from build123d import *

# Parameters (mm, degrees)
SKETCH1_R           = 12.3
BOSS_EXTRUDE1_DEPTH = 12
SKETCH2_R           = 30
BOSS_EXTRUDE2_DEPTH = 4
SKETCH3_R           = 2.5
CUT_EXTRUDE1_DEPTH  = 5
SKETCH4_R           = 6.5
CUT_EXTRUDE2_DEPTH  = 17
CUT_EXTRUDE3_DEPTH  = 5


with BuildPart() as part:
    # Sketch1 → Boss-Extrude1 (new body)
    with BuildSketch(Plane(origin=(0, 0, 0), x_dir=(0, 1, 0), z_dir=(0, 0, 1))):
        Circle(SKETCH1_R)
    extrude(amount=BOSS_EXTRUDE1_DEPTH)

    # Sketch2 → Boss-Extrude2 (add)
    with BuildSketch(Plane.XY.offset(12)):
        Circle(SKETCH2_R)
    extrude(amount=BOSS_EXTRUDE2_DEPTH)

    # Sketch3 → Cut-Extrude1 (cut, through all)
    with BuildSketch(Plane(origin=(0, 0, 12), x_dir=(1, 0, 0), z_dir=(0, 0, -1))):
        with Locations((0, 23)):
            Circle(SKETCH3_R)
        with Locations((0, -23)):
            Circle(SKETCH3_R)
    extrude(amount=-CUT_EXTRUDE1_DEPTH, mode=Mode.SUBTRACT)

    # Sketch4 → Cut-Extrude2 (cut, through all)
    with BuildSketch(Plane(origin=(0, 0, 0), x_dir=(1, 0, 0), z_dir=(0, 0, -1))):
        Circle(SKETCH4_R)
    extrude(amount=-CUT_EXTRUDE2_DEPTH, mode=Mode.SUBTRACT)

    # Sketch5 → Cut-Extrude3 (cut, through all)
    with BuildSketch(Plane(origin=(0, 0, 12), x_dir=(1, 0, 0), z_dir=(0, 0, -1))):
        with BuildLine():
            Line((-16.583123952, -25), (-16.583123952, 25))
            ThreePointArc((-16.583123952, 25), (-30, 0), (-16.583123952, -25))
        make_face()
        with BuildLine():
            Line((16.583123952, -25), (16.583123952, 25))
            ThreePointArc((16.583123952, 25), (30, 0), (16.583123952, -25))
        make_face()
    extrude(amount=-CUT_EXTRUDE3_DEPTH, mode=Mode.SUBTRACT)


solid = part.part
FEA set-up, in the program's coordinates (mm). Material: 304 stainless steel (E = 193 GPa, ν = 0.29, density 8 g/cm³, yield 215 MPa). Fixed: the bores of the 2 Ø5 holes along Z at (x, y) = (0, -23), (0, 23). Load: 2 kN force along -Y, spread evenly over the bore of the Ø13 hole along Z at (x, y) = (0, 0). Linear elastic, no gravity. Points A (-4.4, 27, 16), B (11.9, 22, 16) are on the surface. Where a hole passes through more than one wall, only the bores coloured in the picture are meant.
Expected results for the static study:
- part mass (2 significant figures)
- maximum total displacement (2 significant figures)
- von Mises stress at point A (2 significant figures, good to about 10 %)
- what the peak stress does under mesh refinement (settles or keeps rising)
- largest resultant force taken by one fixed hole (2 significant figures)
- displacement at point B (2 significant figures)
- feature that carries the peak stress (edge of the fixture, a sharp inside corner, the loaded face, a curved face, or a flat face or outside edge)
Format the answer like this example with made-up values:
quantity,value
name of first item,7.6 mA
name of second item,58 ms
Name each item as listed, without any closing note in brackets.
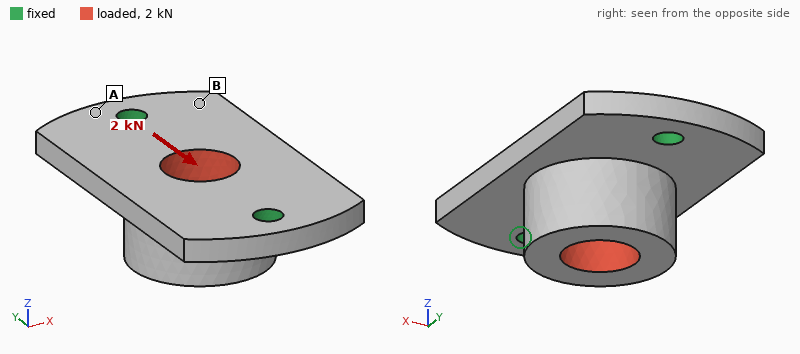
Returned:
quantity,value
part mass,88 g
maximum total displacement,5.2 µm
von Mises stress at point A,12 MPa
what the peak stress does under mesh refinement,keeps rising
largest resultant force taken by one fixed hole,1.1 kN
displacement at point B,1.3 µm
feature that carries the peak stress,edge of the fixture
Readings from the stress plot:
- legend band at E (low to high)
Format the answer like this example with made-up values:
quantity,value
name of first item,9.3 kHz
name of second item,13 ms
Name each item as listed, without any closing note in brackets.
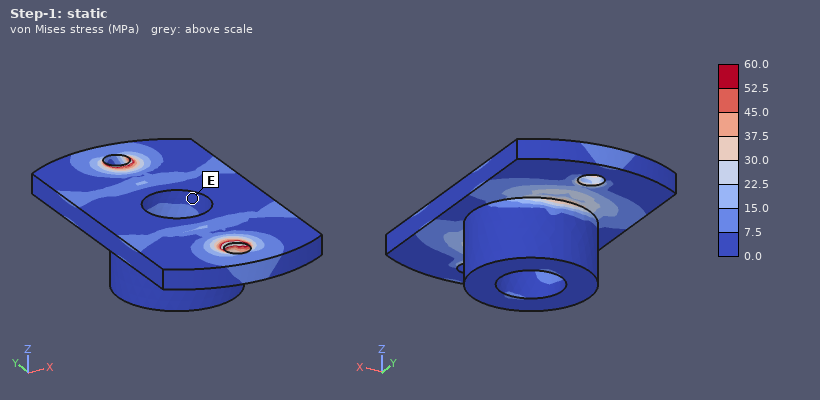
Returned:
quantity,value
legend band at E,0.0 to 7.5 MPa
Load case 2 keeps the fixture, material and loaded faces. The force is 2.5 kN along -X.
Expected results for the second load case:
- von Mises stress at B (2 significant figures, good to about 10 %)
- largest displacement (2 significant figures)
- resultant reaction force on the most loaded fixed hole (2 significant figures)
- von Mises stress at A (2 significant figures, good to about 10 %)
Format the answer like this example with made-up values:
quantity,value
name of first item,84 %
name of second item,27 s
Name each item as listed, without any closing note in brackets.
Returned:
quantity,value
von Mises stress at B,22 MPa
largest displacement,40 µm
resultant reaction force on the most loaded fixed hole,1.3 kN
von Mises stress at A,53 MPa
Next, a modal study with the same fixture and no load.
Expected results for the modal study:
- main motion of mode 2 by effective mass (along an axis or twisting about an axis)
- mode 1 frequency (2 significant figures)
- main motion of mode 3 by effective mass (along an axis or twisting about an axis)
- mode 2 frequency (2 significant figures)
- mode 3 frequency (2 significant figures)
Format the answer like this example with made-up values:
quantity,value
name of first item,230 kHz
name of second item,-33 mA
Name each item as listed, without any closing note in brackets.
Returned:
quantity,value
main motion of mode 2 by effective mass,along Z
mode 1 frequency,5100 Hz
main motion of mode 3 by effective mass,along Y
mode 2 frequency,8200 Hz
mode 3 frequency,14 kHz
